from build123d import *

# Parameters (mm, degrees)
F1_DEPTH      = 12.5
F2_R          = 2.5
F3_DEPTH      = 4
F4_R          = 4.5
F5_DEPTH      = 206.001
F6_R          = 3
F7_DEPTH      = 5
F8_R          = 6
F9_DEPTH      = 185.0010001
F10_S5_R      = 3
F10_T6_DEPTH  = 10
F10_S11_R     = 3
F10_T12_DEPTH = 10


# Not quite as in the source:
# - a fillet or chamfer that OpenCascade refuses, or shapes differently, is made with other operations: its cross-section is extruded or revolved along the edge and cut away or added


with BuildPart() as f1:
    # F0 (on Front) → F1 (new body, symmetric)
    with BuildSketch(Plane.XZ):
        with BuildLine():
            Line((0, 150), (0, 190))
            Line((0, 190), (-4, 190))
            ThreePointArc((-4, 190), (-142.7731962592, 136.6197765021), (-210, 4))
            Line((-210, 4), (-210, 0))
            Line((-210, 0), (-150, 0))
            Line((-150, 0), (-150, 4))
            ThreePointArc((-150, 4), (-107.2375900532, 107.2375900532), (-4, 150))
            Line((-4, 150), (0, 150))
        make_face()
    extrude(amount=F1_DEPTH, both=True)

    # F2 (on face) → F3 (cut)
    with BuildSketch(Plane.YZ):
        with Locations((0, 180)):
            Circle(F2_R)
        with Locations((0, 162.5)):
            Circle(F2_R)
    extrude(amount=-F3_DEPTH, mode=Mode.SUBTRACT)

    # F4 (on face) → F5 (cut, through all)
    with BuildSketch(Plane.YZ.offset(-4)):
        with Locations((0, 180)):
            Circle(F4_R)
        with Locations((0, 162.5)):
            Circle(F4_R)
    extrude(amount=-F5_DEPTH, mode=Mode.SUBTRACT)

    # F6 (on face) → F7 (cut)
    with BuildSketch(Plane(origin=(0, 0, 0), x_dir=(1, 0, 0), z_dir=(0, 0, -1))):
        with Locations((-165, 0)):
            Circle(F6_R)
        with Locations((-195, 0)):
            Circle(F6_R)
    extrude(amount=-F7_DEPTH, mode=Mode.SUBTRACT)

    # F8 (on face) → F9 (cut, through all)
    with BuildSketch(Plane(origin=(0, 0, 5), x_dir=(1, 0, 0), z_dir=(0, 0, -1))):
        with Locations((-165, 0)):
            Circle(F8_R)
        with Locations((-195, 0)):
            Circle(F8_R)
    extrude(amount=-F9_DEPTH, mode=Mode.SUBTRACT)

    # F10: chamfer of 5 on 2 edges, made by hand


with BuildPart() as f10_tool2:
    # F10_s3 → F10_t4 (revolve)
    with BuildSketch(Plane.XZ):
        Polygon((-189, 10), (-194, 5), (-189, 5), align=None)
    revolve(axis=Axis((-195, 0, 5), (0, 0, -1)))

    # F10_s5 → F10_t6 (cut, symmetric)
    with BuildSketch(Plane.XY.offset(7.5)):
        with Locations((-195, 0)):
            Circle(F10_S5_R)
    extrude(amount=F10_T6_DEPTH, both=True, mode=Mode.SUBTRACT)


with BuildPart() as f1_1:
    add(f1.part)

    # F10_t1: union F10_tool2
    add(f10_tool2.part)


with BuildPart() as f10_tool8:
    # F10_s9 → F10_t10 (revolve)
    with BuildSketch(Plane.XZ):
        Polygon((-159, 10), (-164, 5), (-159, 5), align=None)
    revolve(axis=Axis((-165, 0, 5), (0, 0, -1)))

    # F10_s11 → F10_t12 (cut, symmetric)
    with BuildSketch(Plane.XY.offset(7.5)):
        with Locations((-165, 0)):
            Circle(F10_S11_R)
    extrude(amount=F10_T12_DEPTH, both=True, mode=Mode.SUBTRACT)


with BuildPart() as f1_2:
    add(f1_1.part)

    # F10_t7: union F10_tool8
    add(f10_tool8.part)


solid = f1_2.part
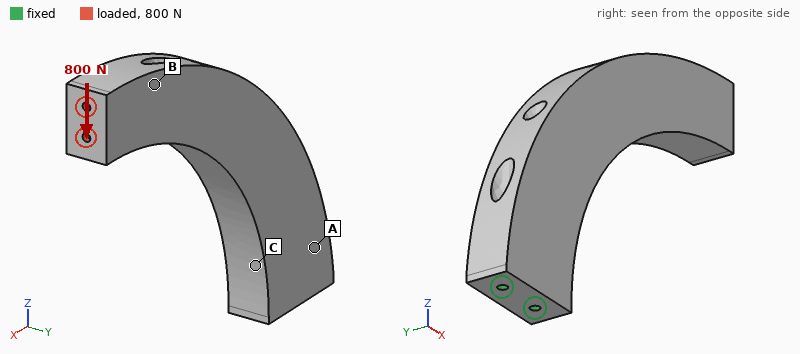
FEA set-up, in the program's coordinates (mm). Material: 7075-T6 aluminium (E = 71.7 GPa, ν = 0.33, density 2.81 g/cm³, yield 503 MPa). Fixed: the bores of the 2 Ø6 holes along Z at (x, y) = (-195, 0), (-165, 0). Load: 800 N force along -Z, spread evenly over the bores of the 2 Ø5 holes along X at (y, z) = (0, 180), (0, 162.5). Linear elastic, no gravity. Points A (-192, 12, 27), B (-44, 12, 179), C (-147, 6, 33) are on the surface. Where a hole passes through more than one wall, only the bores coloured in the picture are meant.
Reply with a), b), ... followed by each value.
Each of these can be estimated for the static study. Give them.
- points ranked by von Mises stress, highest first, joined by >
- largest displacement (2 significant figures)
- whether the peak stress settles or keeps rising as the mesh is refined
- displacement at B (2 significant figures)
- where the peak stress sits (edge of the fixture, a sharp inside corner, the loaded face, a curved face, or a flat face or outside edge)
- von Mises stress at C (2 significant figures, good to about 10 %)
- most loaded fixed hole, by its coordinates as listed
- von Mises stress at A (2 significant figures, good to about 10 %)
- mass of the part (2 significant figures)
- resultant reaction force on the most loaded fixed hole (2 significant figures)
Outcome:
a) C > A > B
b) 0.32 mm
c) keeps rising
d) 0.24 mm
e) edge of the fixture
f) 14 MPa
g) (-165, 0)
h) 8.6 MPa
i) 830 g
j) 4.6 kN
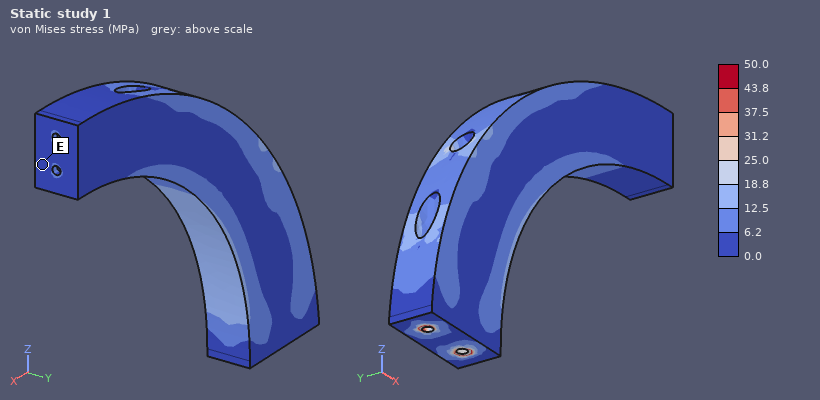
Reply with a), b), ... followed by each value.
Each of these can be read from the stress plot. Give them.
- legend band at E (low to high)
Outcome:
a) 0.0 to 6.2 MPa
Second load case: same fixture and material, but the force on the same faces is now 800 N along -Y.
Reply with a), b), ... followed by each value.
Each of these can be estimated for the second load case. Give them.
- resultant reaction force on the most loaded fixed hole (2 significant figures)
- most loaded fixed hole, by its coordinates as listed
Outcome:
a) 4.4 kN
b) (-165, 0)
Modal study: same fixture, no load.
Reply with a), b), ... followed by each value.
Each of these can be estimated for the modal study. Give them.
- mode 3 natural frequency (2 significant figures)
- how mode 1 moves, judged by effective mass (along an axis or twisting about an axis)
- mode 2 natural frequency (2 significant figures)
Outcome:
a) 1000 Hz
b) along Y
c) 530 Hz
